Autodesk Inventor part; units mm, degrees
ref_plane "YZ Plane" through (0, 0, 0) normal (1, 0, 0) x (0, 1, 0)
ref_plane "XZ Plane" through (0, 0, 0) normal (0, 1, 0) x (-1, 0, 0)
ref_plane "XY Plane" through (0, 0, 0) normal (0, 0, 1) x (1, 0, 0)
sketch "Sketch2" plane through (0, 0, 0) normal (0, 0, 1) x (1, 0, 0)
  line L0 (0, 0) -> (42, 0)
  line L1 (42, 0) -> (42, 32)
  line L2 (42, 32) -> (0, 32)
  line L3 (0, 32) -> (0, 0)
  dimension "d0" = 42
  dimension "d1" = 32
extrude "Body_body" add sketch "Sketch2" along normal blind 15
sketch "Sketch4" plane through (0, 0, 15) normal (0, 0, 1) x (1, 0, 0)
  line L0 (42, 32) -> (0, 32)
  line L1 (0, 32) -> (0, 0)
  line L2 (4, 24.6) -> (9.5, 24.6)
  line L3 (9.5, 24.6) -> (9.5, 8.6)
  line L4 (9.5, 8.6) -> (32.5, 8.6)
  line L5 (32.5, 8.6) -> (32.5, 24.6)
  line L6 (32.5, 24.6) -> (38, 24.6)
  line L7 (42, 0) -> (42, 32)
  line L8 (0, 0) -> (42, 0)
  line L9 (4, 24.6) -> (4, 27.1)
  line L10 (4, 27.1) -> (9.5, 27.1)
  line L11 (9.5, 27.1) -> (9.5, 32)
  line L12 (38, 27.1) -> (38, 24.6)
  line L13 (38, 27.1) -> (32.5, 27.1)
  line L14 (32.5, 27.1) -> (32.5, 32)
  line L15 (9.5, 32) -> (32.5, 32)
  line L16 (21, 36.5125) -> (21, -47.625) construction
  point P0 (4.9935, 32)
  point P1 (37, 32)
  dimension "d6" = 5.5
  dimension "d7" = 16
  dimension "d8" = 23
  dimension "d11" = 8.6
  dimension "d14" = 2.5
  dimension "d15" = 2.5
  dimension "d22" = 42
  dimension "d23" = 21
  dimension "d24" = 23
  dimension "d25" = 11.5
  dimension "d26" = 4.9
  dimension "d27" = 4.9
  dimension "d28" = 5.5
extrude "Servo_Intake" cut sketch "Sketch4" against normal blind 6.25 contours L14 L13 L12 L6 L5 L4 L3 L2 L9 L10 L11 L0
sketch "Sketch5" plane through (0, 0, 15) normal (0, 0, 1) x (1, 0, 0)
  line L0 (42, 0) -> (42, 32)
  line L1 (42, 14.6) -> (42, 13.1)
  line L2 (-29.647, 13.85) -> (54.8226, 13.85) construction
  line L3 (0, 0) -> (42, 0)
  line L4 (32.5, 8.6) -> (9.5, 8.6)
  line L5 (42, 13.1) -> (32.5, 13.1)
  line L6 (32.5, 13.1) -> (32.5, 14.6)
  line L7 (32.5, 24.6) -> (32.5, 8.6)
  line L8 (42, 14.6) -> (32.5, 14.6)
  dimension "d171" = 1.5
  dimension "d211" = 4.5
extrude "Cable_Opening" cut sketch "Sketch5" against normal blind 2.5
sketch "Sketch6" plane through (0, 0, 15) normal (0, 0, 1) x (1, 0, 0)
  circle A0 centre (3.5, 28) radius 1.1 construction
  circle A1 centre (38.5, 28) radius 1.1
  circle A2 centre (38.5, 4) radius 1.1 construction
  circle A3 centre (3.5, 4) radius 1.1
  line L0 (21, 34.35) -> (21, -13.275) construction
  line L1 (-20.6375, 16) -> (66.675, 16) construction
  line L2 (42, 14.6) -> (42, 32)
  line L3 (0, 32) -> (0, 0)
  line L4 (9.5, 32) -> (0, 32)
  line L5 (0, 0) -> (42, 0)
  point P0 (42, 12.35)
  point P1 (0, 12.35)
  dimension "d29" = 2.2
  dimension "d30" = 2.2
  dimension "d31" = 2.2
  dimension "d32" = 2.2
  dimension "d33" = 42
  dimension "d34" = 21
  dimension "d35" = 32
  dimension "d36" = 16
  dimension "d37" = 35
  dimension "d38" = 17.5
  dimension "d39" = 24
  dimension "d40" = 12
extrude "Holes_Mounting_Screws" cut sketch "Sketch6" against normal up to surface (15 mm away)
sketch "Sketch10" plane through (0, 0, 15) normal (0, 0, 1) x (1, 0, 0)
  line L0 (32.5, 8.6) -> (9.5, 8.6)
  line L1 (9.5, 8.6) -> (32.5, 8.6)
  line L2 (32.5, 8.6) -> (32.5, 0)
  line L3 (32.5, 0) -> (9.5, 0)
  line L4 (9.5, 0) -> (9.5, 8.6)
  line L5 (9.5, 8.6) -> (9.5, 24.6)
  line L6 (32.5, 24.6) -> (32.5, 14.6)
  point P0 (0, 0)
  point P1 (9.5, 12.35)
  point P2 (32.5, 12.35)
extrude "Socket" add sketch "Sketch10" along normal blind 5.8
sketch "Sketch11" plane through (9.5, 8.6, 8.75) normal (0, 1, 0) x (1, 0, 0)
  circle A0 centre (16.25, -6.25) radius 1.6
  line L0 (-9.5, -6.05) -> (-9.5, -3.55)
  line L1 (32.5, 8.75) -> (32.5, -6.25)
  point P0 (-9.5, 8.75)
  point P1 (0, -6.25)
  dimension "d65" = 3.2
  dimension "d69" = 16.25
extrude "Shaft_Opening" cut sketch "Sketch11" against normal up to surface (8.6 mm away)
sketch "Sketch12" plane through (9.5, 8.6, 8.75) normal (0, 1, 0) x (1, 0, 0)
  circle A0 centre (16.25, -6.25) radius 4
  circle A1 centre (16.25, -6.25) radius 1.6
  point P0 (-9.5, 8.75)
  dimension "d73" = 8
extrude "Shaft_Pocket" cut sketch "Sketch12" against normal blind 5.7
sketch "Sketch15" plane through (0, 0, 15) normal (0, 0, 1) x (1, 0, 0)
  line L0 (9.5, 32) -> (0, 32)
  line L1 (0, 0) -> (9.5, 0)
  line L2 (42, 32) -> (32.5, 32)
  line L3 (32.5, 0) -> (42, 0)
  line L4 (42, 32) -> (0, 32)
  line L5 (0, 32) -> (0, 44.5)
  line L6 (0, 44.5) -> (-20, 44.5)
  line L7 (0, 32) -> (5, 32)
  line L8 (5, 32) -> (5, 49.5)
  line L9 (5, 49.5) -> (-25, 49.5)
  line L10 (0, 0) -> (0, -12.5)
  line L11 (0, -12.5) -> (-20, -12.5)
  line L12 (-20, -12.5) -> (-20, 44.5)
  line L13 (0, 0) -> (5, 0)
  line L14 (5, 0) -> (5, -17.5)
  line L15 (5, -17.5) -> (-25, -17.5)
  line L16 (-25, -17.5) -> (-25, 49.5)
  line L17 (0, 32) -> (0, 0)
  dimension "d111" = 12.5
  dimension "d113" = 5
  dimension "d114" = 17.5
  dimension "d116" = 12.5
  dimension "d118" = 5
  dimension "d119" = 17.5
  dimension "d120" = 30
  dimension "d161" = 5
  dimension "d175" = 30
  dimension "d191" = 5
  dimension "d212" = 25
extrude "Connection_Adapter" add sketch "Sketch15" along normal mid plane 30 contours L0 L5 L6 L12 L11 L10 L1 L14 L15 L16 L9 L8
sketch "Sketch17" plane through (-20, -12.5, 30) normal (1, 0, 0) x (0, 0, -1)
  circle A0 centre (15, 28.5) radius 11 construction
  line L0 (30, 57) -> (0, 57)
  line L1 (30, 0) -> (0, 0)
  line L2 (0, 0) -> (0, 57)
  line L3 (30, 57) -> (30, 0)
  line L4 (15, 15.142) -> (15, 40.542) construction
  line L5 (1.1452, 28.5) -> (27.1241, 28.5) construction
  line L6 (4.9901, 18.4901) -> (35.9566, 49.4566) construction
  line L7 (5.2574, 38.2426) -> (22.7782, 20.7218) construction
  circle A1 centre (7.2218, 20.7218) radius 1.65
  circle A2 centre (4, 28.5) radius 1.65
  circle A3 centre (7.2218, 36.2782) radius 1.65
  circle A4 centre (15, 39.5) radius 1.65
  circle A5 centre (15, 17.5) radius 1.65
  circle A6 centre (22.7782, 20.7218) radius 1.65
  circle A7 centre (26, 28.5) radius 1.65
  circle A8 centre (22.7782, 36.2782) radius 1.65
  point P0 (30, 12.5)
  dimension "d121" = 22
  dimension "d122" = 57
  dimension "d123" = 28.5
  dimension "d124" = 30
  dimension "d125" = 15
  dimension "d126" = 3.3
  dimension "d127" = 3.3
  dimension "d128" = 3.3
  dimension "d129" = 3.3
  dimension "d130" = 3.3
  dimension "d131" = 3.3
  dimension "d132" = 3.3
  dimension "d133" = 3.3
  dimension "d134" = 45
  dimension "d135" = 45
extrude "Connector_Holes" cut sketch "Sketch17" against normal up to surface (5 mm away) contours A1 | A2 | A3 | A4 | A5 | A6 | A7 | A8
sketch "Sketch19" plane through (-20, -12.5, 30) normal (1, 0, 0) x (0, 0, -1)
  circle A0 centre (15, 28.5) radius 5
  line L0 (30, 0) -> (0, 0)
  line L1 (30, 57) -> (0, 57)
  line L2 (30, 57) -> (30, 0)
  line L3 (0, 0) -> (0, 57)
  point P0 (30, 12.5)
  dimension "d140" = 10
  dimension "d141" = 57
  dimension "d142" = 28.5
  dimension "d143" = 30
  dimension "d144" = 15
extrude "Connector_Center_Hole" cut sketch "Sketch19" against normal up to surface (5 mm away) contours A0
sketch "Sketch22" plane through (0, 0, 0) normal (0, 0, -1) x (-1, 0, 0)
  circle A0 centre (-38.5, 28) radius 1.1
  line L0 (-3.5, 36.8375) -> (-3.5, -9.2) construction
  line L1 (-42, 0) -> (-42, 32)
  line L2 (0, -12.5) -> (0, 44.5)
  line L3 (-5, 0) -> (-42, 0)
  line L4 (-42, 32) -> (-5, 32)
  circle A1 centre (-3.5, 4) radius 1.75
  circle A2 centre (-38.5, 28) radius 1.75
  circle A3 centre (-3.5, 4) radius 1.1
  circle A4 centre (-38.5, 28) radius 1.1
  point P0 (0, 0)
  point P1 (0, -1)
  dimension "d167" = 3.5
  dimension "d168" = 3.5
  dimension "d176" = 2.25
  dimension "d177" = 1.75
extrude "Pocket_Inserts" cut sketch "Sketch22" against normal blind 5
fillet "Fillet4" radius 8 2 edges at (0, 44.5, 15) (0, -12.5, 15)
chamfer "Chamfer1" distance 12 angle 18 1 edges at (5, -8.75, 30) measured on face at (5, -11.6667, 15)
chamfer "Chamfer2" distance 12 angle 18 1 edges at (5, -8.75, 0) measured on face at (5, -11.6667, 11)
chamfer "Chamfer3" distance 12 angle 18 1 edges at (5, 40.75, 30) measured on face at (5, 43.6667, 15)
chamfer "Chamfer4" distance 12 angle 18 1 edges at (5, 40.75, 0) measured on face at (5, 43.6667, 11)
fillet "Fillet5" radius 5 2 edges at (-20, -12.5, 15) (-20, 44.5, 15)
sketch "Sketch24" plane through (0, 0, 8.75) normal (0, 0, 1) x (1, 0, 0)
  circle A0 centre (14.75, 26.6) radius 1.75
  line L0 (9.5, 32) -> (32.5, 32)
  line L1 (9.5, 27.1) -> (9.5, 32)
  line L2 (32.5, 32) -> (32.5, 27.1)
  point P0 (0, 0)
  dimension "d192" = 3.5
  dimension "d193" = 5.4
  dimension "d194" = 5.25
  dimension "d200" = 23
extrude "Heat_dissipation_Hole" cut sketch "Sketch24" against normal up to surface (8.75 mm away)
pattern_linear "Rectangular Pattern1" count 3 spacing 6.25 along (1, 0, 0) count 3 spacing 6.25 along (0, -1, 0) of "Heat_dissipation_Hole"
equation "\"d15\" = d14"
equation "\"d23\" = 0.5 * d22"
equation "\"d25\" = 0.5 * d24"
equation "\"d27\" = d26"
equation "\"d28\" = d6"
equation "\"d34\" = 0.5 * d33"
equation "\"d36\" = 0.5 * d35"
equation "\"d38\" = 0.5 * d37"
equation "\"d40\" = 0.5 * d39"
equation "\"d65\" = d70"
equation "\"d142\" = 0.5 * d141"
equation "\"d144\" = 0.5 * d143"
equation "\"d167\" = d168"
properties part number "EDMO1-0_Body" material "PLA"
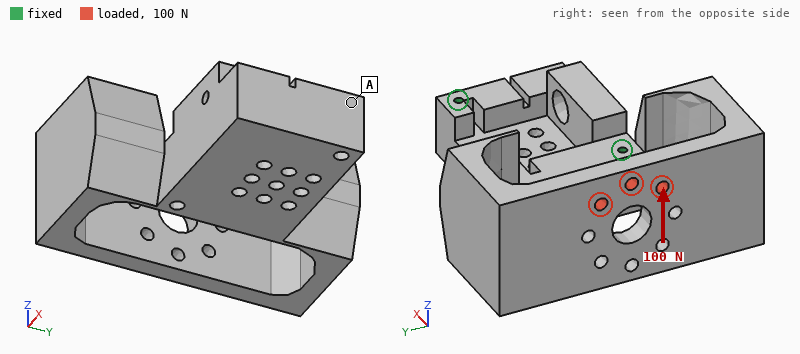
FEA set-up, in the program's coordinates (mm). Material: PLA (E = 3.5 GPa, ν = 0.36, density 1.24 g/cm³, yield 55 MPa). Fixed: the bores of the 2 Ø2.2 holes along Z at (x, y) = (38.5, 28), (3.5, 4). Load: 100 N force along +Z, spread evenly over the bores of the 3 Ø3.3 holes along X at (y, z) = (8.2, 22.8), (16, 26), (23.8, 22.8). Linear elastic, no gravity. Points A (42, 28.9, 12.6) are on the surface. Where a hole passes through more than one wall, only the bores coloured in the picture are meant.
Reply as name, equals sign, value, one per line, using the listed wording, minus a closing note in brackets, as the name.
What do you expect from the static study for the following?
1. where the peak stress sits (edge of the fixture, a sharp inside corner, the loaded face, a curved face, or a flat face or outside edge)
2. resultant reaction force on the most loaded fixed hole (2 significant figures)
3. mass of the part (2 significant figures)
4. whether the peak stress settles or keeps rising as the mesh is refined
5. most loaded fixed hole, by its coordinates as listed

where the peak stress sits = edge of the fixture
resultant reaction force on the most loaded fixed hole = 130 N
mass of the part = 45 g
whether the peak stress settles or keeps rising as the mesh is refined = keeps rising
most loaded fixed hole, by its coordinates as listed = (3.5, 4)
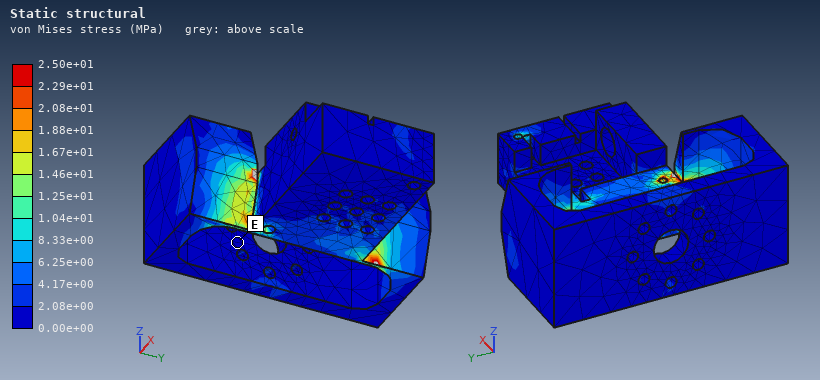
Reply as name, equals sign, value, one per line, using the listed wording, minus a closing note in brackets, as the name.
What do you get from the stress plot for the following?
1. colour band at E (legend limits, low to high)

colour band at E = 0.00e+00 to 2.08e+00 MPa
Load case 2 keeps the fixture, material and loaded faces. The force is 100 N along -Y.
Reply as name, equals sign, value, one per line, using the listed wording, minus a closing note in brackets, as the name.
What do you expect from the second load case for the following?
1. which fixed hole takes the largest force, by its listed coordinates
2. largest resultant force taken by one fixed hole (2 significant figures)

which fixed hole takes the largest force, by its listed coordinates = (3.5, 4)
largest resultant force taken by one fixed hole = 150 N
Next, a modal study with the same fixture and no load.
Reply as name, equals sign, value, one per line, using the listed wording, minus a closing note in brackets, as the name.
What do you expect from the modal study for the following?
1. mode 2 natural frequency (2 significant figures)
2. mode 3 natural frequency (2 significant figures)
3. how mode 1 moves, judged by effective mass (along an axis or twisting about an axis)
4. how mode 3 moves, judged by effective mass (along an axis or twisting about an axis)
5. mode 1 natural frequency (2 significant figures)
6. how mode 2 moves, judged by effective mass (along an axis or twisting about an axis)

mode 2 natural frequency = 500 Hz
mode 3 natural frequency = 820 Hz
how mode 1 moves, judged by effective mass = along Z
how mode 3 moves, judged by effective mass = twisting about X
mode 1 natural frequency = 430 Hz
how mode 2 moves, judged by effective mass = along Y
